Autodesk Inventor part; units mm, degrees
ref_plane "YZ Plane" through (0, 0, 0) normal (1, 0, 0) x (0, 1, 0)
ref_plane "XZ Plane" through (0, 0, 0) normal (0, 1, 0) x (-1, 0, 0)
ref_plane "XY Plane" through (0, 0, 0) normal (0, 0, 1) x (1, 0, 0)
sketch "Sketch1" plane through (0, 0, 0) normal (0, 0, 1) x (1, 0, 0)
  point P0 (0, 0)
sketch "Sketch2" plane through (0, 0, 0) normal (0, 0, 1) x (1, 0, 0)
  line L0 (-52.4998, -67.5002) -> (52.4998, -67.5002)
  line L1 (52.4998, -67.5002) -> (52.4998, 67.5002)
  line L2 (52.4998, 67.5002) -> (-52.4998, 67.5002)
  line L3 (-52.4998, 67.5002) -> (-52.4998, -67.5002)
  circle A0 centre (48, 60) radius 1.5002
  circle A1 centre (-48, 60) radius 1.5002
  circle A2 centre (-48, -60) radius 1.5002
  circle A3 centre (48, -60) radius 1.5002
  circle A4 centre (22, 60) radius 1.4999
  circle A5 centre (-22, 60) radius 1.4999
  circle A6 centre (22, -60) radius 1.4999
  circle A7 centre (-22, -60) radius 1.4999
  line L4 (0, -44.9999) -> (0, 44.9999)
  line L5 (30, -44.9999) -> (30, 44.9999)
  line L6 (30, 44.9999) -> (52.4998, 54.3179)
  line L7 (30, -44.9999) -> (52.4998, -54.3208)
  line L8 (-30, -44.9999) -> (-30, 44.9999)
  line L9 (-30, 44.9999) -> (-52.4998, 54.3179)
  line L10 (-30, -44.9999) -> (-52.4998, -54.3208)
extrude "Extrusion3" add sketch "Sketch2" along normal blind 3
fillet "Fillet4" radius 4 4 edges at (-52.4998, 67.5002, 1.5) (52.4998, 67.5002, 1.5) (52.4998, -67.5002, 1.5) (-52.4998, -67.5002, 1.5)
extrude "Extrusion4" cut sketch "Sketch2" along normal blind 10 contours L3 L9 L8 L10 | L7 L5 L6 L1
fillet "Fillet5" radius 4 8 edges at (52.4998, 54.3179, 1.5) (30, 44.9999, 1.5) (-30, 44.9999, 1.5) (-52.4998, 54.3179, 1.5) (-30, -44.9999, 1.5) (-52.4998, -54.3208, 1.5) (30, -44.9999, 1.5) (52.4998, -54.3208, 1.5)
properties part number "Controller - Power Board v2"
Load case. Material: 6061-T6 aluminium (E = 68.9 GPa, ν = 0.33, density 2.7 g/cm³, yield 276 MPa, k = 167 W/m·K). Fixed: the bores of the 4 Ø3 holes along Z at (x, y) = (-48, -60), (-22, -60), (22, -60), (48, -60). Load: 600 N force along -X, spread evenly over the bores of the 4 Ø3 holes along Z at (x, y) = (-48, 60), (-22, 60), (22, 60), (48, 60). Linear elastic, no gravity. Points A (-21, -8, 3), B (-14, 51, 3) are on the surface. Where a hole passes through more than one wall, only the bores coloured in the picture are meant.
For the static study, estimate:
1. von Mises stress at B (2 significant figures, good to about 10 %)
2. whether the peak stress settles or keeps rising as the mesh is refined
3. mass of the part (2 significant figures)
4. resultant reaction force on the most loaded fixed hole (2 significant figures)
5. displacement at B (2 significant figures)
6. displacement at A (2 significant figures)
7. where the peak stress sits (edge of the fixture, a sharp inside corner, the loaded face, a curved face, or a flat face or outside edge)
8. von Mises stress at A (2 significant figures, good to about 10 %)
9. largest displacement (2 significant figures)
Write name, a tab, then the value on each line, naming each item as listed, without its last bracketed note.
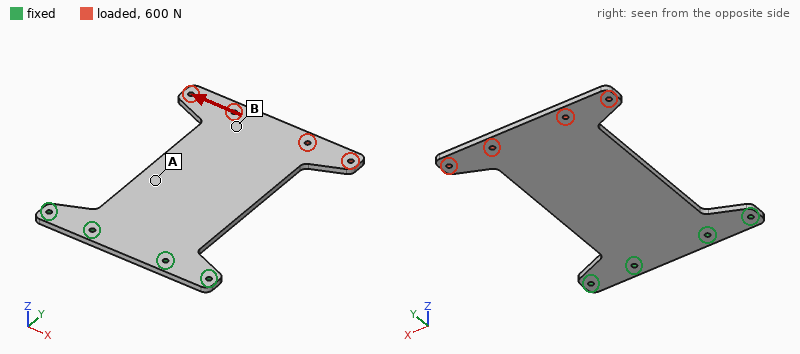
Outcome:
von Mises stress at B	6.9 MPa
whether the peak stress settles or keeps rising as the mesh is refined	keeps rising
mass of the part	78 g
resultant reaction force on the most loaded fixed hole	1.1 kN
displacement at B	0.095 mm
displacement at A	0.031 mm
where the peak stress sits	edge of the fixture
von Mises stress at A	17 MPa
largest displacement	0.13 mm
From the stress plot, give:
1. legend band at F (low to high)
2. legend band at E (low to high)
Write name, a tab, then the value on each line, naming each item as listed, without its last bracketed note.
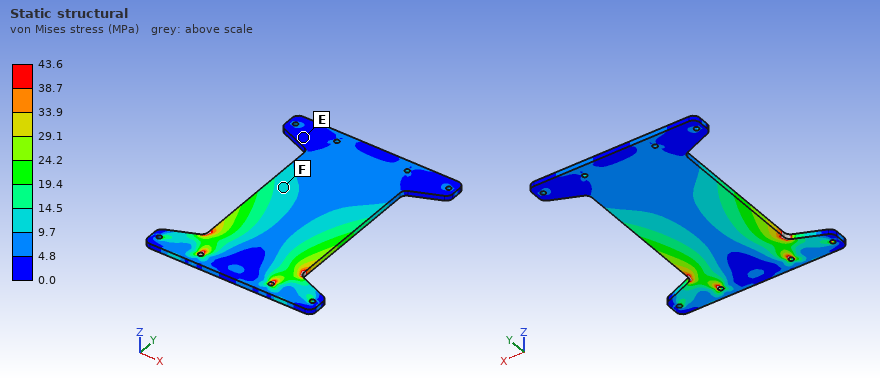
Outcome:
legend band at F	9.7 to 14.5 MPa
legend band at E	0.0 to 4.8 MPa
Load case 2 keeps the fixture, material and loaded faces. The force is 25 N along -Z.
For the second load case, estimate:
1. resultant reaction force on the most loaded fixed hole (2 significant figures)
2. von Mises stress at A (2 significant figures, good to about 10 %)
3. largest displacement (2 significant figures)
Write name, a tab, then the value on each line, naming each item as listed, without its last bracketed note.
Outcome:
resultant reaction force on the most loaded fixed hole	22 N
von Mises stress at A	19 MPa
largest displacement	1.7 mm
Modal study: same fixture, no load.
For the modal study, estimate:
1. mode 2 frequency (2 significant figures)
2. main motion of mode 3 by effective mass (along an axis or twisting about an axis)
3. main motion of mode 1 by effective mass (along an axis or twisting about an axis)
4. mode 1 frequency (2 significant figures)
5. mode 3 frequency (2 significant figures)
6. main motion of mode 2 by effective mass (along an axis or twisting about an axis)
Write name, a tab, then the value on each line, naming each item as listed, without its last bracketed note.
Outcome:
mode 2 frequency	460 Hz
main motion of mode 3 by effective mass	along Z
main motion of mode 1 by effective mass	along Z
mode 1 frequency	130 Hz
mode 3 frequency	880 Hz
main motion of mode 2 by effective mass	twisting about Y
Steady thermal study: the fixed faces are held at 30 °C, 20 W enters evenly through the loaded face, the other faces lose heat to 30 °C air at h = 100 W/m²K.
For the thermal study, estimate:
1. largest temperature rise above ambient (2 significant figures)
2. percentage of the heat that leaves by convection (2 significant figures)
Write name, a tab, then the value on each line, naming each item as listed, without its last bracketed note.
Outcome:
largest temperature rise above ambient	31 K
percentage of the heat that leaves by convection	90 %
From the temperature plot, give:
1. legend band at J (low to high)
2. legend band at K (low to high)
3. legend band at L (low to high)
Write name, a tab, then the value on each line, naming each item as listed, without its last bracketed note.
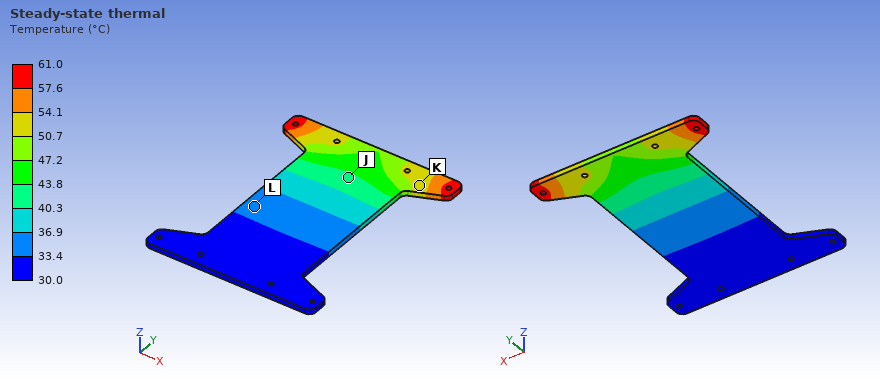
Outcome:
legend band at J	40.3 to 43.8 °C
legend band at K	50.7 to 54.1 °C
legend band at L	33.4 to 36.9 °C
